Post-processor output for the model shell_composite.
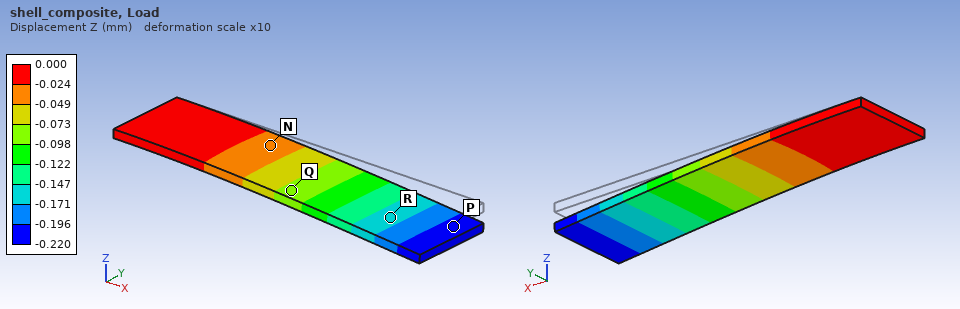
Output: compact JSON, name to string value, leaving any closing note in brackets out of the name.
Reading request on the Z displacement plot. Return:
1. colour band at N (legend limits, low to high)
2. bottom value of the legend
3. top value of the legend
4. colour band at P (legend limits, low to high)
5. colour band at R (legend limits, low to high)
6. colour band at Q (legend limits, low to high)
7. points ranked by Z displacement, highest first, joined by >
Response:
{"colour band at N": "-0.049 to -0.024 mm", "bottom value of the legend": "-0.220 mm", "top value of the legend": "0.000 mm", "colour band at P": "-0.220 to -0.196 mm", "colour band at R": "-0.171 to -0.147 mm", "colour band at Q": "-0.098 to -0.073 mm", "points ranked by Z displacement, highest first, joined by >": "N > Q > R > P"}
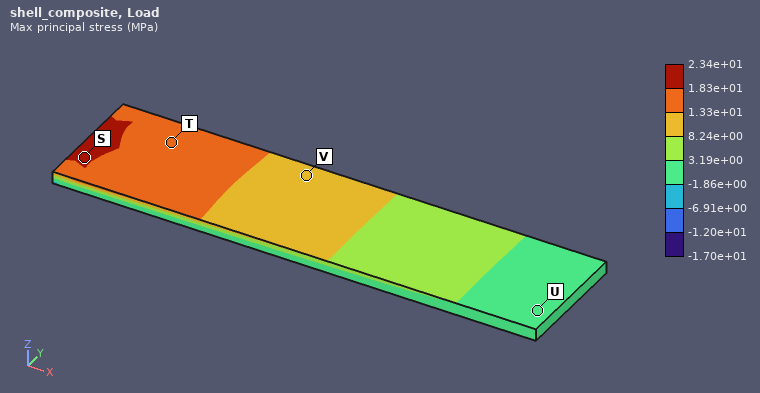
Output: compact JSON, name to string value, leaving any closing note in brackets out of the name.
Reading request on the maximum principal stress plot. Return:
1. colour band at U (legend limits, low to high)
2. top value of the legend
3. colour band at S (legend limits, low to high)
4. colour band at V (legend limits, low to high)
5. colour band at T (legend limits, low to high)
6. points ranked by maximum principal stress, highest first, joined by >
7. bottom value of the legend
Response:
{"colour band at U": "-1.86e+00 to 3.19e+00 MPa", "top value of the legend": "2.34e+01 MPa", "colour band at S": "1.83e+01 to 2.34e+01 MPa", "colour band at V": "8.24e+00 to 1.33e+01 MPa", "colour band at T": "1.33e+01 to 1.83e+01 MPa", "points ranked by maximum principal stress, highest first, joined by >": "S > T > V > U", "bottom value of the legend": "-1.70e+01 MPa"}
